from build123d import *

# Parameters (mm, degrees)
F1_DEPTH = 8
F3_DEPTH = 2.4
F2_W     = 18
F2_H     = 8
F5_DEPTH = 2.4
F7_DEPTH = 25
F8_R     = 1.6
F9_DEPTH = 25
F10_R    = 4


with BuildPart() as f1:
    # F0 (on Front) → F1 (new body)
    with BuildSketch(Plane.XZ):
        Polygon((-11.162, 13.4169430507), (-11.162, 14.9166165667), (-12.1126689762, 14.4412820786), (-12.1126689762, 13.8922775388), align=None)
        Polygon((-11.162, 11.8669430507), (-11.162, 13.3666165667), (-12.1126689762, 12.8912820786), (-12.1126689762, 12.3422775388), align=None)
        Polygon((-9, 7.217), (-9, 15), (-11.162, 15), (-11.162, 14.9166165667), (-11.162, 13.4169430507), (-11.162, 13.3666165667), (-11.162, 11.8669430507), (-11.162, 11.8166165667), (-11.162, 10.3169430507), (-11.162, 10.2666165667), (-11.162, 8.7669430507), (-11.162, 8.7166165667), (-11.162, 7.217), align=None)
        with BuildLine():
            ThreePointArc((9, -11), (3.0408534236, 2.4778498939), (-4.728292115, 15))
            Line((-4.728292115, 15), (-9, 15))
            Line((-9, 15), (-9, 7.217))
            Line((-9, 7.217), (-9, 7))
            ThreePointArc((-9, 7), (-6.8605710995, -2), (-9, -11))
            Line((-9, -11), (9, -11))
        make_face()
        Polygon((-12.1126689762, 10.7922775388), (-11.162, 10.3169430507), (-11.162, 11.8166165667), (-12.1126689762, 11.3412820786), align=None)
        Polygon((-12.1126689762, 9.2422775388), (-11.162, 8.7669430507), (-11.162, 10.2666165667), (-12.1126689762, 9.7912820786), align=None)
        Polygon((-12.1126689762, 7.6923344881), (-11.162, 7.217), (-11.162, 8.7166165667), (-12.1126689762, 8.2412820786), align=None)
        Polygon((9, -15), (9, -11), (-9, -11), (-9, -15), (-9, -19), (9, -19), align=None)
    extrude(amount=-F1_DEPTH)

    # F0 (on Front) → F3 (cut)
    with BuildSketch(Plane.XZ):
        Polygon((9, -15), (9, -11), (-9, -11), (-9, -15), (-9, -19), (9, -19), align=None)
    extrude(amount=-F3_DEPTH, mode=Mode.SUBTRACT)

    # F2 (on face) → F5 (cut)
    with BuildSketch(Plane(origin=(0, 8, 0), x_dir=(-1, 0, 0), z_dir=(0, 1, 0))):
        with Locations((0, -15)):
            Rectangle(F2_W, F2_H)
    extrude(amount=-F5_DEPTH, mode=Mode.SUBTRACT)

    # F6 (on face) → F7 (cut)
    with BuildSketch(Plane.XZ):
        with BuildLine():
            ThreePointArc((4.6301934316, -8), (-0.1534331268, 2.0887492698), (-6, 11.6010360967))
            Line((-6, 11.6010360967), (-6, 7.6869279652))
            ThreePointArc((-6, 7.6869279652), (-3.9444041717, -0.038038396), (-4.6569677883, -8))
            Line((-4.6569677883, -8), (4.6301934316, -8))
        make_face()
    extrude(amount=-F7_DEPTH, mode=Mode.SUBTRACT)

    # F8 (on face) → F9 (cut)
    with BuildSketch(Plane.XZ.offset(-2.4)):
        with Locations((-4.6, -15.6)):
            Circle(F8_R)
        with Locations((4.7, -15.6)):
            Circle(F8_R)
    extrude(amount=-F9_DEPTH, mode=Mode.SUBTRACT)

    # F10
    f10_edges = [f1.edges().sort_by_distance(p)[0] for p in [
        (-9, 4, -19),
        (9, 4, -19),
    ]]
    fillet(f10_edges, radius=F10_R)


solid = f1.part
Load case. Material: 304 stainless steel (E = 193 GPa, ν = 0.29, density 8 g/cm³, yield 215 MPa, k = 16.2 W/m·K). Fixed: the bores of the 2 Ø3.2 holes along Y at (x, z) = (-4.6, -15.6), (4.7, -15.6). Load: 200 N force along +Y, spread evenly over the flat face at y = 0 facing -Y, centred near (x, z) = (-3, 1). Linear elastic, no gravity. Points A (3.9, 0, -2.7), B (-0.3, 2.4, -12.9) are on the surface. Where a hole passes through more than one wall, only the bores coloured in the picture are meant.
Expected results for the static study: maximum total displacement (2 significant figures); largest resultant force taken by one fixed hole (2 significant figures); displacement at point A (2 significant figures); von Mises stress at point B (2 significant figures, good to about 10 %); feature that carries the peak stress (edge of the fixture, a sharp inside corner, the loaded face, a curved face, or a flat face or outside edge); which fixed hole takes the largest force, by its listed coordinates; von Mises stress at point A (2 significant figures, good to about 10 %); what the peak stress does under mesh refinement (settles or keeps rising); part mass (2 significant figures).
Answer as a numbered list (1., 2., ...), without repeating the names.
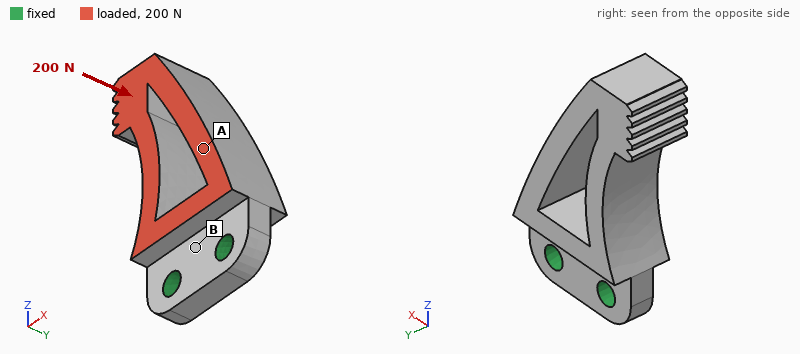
1. 52 µm
2. 140 N
3. 16 µm
4. 59 MPa
5. edge of the fixture
6. (-4.6, -15.6)
7. 21 MPa
8. keeps rising
9. 17 g
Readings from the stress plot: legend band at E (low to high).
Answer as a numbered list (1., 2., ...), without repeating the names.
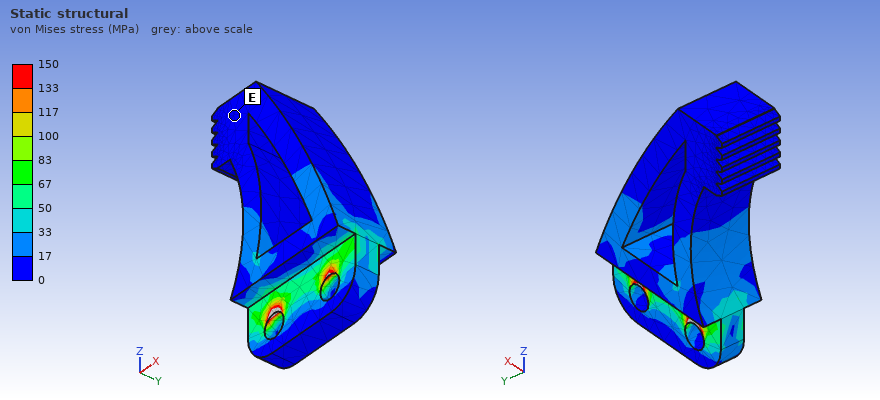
1. 0 to 17 MPa
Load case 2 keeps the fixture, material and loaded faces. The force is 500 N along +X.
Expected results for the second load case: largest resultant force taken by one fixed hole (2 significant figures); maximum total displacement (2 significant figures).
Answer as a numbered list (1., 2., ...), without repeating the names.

1. 750 N
2. 28 µm
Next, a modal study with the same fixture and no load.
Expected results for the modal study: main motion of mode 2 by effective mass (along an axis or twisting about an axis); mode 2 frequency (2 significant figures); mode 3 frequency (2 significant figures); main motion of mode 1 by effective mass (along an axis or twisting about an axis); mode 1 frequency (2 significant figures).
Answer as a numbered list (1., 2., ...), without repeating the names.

1. along X
2. 7600 Hz
3. 13 kHz
4. along Y
5. 3200 Hz
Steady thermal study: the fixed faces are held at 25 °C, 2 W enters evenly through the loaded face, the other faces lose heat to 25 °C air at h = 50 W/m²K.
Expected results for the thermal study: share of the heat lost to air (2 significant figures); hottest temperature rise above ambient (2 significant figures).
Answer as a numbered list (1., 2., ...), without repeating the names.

1. 45 %
2. 21 K
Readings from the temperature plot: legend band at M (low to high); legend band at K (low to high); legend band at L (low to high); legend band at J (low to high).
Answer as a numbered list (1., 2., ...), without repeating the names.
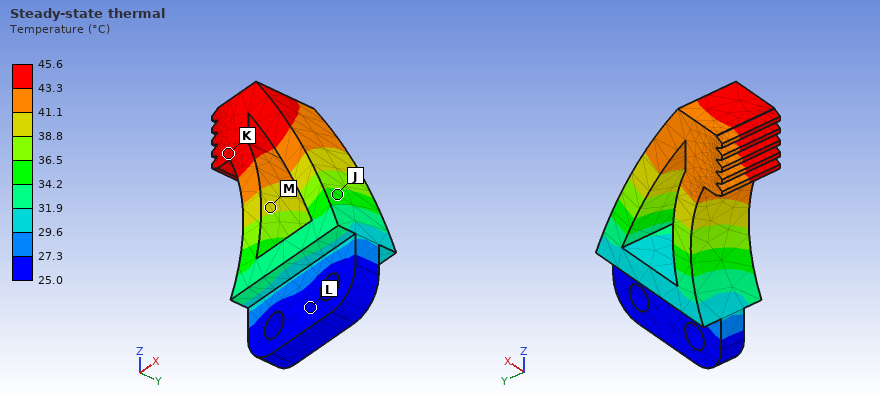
1. 38.8 to 41.1 °C
2. 43.3 to 45.6 °C
3. 25.0 to 27.3 °C
4. 34.2 to 36.5 °C
